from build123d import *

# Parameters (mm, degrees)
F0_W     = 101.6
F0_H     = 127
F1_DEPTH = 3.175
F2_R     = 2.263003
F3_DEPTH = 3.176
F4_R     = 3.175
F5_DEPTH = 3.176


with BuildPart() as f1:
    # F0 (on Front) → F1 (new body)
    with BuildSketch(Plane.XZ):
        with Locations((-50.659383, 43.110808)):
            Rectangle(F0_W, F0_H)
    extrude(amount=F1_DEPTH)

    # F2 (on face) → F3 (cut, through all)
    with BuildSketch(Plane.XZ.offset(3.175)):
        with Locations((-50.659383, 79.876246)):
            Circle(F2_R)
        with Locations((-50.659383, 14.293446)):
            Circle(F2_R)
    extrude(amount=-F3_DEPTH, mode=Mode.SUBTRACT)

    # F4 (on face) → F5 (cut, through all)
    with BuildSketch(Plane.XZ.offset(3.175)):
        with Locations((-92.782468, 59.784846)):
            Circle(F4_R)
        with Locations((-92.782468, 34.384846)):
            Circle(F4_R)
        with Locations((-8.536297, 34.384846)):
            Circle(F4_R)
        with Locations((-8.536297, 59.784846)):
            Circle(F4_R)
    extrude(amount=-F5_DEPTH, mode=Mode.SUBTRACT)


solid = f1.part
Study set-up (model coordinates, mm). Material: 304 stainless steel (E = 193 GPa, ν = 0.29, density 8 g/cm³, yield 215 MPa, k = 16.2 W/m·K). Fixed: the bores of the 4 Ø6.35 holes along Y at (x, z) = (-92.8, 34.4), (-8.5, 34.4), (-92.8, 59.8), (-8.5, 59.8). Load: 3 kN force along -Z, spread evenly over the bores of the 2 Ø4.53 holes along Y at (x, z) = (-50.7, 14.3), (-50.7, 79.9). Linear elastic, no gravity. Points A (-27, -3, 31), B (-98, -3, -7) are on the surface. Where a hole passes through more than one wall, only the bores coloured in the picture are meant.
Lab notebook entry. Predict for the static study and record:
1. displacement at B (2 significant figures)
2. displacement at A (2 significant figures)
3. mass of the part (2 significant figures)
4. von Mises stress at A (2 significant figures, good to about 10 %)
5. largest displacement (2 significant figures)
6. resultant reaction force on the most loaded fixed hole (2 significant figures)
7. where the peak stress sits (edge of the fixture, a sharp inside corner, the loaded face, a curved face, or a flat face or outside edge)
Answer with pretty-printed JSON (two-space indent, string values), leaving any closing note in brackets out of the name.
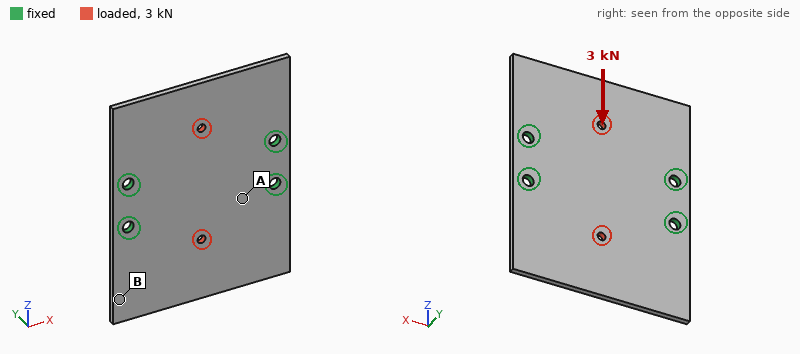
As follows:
{
  "displacement at B": "0.95 µm",
  "displacement at A": "1.6 µm",
  "mass of the part": "320 g",
  "von Mises stress at A": "8.3 MPa",
  "largest displacement": "4.1 µm",
  "resultant reaction force on the most loaded fixed hole": "770 N",
  "where the peak stress sits": "the loaded face"
}
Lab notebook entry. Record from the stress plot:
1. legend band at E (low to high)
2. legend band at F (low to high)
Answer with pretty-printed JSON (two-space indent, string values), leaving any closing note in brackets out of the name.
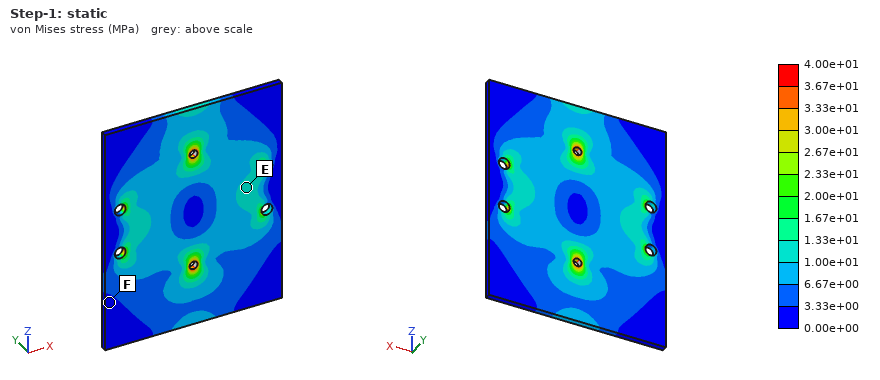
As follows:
{
  "legend band at E": "1.00e+01 to 1.33e+01 MPa",
  "legend band at F": "0.00e+00 to 3.33e+00 MPa"
}
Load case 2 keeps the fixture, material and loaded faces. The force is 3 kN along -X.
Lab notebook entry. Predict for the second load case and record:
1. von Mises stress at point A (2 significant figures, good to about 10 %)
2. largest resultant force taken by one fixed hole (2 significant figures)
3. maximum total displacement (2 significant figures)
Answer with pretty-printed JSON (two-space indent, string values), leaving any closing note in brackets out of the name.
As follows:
{
  "von Mises stress at point A": "8.8 MPa",
  "largest resultant force taken by one fixed hole": "770 N",
  "maximum total displacement": "3.5 µm"
}
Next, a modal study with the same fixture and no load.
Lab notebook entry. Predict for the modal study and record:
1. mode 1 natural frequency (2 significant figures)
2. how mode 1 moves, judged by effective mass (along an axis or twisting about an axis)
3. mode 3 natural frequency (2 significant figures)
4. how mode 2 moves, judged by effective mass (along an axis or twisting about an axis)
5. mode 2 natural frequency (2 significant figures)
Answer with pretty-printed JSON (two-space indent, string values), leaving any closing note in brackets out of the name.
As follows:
{
  "mode 1 natural frequency": "730 Hz",
  "how mode 1 moves, judged by effective mass": "along Y",
  "mode 3 natural frequency": "1400 Hz",
  "how mode 2 moves, judged by effective mass": "along Y",
  "mode 2 natural frequency": "960 Hz"
}
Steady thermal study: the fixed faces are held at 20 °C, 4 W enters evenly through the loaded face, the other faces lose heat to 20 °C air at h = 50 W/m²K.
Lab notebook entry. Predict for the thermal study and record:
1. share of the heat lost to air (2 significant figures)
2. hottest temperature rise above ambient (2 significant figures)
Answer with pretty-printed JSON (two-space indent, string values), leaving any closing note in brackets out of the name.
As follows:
{
  "share of the heat lost to air": "85 %",
  "hottest temperature rise above ambient": "16 K"
}
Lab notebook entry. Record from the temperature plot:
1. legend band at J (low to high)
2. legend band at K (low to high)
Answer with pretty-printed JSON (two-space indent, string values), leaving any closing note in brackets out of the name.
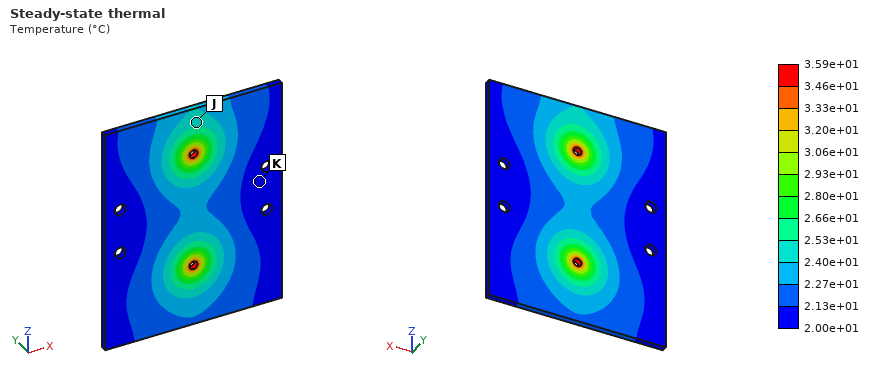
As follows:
{
  "legend band at J": "2.40e+01 to 2.53e+01 °C",
  "legend band at K": "2.00e+01 to 2.13e+01 °C"
}
